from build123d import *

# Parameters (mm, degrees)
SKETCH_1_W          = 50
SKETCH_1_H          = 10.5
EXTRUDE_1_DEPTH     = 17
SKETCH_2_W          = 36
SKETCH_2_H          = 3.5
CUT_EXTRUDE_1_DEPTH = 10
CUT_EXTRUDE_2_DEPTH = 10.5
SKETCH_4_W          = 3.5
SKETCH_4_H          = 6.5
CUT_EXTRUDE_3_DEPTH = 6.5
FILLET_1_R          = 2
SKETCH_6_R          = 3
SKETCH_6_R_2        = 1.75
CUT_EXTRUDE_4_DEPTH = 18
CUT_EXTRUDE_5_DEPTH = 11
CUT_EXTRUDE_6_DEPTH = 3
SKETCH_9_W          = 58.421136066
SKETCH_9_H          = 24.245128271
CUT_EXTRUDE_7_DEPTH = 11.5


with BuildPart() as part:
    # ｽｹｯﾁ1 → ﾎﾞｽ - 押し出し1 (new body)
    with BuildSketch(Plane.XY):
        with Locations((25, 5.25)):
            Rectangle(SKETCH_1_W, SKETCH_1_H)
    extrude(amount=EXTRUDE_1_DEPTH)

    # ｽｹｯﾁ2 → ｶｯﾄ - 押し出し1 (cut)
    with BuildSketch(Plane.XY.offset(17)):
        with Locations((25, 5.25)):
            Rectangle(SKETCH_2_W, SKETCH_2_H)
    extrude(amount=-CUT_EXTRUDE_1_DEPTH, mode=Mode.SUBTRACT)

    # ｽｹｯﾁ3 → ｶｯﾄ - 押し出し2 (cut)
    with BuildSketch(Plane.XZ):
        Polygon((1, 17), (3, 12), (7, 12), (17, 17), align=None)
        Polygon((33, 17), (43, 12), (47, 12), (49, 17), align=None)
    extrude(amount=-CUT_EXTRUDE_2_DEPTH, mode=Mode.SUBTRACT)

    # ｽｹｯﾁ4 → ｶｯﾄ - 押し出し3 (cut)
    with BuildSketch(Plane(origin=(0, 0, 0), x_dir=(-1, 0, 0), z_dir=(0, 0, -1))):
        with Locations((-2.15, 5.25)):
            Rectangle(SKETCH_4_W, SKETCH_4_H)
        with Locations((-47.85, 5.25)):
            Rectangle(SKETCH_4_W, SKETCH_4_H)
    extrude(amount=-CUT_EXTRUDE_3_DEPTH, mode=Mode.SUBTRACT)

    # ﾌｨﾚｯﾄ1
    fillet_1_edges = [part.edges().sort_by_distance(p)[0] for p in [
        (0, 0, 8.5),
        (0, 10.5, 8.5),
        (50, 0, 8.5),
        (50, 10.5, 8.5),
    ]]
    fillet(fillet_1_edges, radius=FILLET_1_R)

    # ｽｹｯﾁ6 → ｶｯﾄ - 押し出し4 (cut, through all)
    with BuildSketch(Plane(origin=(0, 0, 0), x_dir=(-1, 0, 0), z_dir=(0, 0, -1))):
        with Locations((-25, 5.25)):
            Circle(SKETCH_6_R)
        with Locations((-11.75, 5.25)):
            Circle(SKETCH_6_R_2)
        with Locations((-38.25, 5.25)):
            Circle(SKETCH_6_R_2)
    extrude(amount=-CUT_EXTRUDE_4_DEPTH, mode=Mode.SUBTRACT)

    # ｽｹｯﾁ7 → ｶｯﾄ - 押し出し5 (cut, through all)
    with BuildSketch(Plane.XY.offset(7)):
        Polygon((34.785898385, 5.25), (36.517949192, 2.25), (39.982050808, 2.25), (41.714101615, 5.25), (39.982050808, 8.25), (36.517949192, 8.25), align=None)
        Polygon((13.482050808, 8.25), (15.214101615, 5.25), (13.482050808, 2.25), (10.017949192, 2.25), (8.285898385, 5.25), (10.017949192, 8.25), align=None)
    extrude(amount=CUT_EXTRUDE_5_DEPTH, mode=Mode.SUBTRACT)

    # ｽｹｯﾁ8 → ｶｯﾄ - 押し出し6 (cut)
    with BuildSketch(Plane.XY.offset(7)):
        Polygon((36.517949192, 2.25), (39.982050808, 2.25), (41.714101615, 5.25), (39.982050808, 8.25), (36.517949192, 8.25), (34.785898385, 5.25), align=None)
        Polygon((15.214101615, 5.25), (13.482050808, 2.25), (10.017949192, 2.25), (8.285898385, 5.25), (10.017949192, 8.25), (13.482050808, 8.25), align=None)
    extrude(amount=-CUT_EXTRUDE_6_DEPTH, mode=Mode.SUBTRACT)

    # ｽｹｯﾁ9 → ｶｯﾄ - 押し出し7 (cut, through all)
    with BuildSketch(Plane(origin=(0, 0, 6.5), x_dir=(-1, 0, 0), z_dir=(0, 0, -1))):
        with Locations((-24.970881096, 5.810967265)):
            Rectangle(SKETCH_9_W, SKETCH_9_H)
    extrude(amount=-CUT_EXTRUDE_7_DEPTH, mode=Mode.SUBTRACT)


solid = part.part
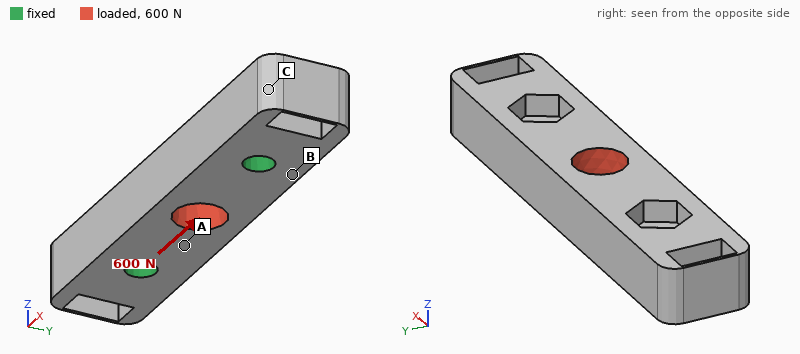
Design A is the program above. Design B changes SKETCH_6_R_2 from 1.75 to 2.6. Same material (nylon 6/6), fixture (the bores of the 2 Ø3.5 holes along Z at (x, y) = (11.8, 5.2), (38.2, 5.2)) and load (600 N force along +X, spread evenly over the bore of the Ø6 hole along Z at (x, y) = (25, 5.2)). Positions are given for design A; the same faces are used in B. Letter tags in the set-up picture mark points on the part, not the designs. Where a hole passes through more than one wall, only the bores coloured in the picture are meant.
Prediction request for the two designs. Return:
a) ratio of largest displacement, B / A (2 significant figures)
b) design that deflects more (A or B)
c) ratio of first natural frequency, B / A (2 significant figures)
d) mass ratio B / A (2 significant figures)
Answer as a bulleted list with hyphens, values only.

- 0.85
- A
- 1.3
- 0.97
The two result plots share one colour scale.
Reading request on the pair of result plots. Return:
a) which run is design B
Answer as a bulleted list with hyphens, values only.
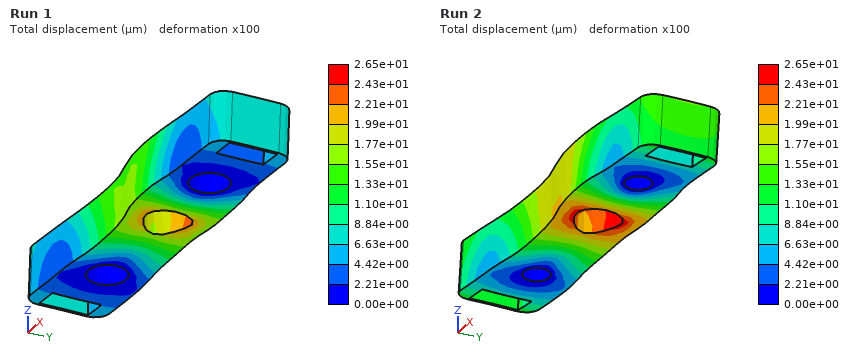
- Run 1
